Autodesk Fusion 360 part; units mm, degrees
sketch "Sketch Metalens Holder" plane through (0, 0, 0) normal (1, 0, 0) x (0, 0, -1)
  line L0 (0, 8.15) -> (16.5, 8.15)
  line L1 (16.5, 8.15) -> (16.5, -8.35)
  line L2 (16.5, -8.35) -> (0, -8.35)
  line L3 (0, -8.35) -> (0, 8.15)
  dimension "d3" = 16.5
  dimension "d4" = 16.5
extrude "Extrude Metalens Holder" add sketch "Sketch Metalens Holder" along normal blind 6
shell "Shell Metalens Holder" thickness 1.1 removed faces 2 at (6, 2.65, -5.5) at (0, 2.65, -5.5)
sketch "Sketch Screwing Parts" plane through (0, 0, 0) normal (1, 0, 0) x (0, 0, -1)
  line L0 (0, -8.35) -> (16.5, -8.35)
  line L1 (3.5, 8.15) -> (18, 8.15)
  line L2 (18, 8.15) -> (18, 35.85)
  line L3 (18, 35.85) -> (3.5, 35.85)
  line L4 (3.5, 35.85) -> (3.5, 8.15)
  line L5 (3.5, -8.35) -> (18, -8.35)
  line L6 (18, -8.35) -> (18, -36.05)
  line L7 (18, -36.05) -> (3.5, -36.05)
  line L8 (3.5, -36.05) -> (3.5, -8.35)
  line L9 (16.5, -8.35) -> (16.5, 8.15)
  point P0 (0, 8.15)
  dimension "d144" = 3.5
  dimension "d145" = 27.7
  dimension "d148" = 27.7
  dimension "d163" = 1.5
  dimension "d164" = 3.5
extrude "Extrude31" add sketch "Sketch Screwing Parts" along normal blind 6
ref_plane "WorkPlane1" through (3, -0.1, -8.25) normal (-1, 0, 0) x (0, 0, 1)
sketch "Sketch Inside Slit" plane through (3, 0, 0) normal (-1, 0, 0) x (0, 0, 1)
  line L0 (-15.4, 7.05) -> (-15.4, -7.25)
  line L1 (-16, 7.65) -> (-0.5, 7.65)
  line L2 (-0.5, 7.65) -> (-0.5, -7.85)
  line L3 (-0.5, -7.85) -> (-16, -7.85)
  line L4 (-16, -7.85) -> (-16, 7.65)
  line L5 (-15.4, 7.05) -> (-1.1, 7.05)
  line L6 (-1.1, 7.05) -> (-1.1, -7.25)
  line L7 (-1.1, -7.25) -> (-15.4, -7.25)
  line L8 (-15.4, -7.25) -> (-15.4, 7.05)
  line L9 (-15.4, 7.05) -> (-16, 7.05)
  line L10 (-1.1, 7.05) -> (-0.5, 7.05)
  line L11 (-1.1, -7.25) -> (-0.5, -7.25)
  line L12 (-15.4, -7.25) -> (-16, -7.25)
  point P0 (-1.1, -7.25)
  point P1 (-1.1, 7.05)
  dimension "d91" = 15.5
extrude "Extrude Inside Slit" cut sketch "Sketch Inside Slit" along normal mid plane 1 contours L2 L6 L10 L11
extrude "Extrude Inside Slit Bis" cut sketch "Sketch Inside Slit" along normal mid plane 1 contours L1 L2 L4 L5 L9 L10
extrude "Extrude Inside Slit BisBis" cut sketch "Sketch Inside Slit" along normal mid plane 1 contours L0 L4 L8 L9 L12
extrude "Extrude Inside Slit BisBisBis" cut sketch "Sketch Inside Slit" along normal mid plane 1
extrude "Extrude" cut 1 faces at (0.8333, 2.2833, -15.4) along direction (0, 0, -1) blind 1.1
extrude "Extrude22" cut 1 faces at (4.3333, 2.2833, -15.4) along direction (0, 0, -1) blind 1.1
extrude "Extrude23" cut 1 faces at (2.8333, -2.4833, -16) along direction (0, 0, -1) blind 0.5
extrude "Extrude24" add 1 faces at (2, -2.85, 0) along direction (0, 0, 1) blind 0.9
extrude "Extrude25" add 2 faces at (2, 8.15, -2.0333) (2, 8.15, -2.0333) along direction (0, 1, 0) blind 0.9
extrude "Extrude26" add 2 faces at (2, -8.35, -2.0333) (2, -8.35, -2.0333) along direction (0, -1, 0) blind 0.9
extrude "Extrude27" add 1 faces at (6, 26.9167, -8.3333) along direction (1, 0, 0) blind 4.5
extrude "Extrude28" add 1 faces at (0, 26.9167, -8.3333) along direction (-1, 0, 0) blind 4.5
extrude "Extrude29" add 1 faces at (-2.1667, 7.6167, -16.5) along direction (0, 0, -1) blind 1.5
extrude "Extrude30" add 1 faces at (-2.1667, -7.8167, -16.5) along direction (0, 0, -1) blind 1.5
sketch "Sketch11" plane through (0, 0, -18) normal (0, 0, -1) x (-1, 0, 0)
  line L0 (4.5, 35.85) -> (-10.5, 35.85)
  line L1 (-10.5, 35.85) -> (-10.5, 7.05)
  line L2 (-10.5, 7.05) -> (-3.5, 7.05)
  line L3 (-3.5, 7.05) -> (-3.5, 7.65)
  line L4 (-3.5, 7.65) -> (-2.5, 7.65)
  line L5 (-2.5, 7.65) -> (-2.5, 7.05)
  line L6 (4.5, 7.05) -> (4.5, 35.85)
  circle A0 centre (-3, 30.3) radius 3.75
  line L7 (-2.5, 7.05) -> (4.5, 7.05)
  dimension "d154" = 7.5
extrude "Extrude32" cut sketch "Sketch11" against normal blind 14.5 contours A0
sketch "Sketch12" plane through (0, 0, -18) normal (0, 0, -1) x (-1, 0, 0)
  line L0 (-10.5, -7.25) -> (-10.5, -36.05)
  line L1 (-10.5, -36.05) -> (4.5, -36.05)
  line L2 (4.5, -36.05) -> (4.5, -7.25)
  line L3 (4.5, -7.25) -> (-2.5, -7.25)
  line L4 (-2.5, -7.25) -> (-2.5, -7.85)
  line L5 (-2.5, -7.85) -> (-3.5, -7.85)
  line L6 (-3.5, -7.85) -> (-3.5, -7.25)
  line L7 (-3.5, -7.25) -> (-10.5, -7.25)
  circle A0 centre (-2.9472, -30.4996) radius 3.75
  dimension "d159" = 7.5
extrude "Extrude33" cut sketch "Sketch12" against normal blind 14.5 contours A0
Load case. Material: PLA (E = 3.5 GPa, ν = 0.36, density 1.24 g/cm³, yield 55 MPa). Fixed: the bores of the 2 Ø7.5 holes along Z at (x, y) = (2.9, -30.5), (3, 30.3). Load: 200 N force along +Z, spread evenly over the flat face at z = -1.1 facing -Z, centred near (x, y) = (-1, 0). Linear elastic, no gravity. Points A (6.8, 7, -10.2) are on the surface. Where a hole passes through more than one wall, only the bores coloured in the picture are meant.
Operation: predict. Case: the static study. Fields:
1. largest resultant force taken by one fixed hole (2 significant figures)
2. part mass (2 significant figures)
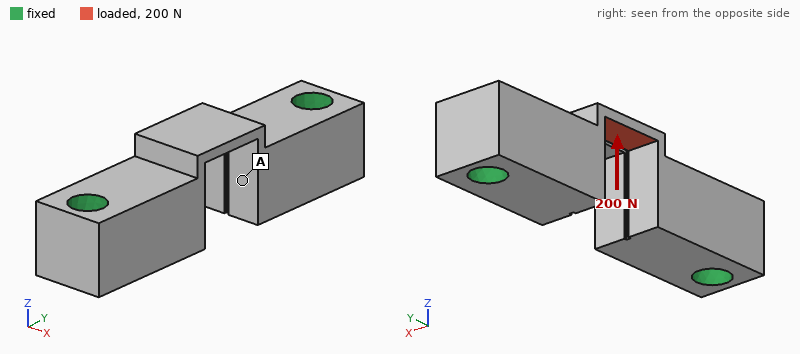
140 N
15 g
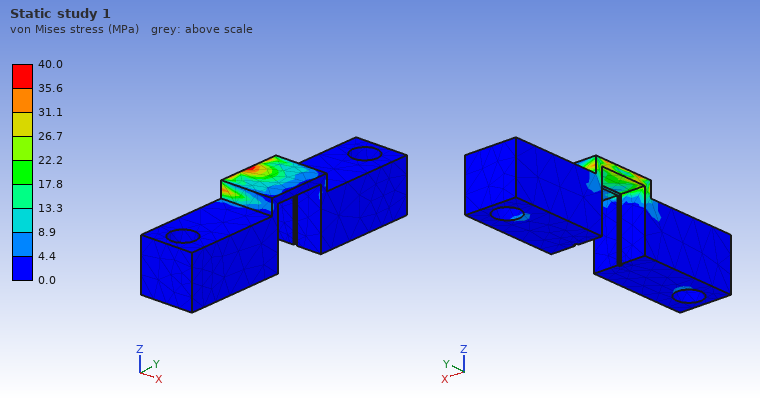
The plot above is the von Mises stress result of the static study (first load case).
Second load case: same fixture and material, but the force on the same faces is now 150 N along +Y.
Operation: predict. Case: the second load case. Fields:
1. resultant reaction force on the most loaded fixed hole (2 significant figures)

78 N
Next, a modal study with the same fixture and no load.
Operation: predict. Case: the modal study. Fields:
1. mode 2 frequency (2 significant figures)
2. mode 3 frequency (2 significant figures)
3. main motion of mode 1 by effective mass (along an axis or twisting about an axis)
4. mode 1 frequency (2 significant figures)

6400 Hz
6400 Hz
along X
5200 Hz
